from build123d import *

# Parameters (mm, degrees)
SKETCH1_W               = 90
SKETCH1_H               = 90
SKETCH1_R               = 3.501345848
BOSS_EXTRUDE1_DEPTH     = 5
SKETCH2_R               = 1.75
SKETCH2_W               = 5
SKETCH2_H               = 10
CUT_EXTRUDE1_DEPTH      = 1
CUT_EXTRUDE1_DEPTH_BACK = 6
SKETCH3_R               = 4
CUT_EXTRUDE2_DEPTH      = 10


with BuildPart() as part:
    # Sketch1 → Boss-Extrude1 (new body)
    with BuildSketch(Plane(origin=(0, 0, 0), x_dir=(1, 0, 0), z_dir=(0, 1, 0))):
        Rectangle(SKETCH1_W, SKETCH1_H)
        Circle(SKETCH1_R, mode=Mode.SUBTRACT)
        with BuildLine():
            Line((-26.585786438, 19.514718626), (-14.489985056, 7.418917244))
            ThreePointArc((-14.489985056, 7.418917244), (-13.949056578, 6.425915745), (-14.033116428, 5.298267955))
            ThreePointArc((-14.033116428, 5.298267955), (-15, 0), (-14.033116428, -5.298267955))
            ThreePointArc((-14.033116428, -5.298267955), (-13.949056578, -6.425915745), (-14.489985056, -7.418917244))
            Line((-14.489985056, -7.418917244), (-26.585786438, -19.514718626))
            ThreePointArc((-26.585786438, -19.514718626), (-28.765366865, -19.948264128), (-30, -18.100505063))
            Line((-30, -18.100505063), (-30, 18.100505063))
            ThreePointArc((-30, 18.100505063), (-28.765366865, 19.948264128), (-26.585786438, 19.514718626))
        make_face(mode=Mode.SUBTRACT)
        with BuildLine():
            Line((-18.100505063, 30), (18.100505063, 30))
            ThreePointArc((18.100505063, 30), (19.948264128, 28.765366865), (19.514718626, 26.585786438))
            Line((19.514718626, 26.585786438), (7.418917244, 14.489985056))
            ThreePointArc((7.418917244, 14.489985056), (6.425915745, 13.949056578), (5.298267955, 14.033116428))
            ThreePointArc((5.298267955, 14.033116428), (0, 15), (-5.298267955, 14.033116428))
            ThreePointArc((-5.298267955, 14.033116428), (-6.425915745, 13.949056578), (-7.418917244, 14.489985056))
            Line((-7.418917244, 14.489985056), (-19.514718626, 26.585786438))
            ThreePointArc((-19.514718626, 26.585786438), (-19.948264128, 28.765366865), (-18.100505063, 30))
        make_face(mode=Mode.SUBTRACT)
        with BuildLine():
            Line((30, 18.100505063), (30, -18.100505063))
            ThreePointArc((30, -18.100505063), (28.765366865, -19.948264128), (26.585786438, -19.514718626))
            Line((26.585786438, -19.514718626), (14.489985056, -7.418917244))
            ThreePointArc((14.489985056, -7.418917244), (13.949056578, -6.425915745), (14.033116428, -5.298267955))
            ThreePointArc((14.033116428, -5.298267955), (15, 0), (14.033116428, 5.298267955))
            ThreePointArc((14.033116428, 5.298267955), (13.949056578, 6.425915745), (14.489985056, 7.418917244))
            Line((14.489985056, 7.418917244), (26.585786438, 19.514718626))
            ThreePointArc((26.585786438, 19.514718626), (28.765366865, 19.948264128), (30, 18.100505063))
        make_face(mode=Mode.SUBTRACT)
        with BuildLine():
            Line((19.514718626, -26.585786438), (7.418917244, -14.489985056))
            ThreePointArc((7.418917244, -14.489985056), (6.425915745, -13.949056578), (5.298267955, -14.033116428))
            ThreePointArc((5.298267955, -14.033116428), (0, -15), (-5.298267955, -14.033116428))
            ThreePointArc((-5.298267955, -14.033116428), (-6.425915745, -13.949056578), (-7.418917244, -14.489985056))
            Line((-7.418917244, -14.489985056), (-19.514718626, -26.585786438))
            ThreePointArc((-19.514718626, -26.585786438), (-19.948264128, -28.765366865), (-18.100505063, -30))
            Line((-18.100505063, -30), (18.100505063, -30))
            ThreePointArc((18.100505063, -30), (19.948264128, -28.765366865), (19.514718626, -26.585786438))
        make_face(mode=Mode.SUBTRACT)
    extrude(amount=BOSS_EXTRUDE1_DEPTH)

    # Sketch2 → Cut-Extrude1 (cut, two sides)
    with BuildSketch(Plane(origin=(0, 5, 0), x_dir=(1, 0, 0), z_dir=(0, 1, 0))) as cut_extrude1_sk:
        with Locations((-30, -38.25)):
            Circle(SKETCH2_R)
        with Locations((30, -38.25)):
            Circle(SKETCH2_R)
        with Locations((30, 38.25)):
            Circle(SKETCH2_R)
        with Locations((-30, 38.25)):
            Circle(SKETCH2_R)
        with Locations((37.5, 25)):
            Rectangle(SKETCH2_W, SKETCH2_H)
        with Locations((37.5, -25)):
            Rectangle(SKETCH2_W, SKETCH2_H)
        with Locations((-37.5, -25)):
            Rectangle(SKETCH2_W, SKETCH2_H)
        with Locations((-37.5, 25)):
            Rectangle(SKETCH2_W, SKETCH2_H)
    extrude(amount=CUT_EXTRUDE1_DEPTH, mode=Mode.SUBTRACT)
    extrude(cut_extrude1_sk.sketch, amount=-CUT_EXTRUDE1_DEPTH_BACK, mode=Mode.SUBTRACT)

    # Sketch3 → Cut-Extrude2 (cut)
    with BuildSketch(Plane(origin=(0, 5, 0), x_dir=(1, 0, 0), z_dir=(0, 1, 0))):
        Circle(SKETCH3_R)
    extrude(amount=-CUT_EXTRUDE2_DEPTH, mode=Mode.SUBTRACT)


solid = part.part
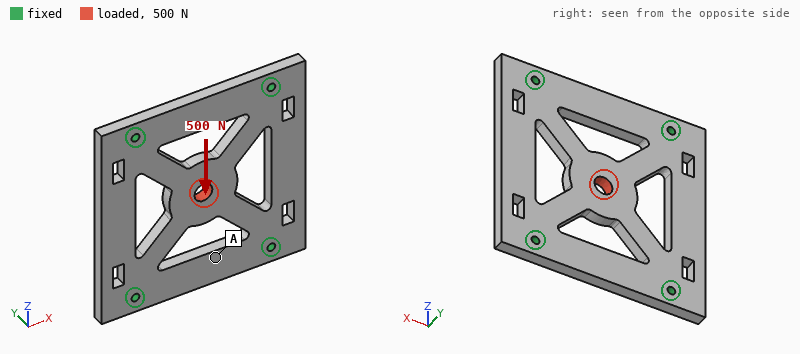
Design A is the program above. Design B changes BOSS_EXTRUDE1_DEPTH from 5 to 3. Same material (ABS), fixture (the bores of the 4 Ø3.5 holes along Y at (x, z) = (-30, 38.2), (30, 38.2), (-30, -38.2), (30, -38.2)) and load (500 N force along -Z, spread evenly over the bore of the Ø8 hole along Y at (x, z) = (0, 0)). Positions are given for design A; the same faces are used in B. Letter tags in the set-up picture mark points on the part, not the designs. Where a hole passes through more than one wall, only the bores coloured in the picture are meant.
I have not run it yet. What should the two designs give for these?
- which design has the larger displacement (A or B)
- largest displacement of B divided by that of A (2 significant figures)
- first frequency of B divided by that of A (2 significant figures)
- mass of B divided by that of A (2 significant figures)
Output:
B
1.7
0.63
0.60
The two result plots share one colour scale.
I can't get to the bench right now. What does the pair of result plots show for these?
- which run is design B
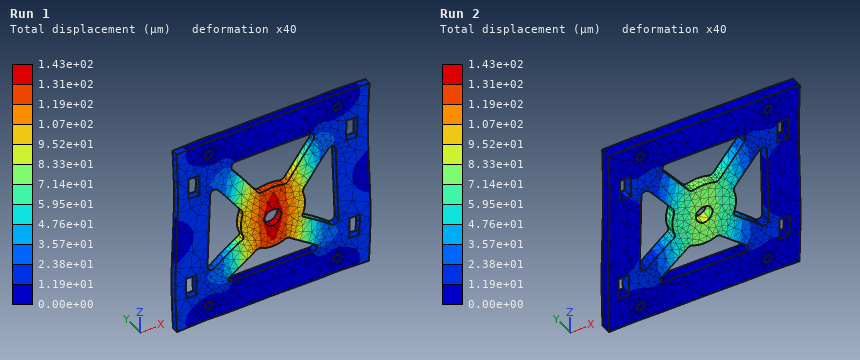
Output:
Run 1
